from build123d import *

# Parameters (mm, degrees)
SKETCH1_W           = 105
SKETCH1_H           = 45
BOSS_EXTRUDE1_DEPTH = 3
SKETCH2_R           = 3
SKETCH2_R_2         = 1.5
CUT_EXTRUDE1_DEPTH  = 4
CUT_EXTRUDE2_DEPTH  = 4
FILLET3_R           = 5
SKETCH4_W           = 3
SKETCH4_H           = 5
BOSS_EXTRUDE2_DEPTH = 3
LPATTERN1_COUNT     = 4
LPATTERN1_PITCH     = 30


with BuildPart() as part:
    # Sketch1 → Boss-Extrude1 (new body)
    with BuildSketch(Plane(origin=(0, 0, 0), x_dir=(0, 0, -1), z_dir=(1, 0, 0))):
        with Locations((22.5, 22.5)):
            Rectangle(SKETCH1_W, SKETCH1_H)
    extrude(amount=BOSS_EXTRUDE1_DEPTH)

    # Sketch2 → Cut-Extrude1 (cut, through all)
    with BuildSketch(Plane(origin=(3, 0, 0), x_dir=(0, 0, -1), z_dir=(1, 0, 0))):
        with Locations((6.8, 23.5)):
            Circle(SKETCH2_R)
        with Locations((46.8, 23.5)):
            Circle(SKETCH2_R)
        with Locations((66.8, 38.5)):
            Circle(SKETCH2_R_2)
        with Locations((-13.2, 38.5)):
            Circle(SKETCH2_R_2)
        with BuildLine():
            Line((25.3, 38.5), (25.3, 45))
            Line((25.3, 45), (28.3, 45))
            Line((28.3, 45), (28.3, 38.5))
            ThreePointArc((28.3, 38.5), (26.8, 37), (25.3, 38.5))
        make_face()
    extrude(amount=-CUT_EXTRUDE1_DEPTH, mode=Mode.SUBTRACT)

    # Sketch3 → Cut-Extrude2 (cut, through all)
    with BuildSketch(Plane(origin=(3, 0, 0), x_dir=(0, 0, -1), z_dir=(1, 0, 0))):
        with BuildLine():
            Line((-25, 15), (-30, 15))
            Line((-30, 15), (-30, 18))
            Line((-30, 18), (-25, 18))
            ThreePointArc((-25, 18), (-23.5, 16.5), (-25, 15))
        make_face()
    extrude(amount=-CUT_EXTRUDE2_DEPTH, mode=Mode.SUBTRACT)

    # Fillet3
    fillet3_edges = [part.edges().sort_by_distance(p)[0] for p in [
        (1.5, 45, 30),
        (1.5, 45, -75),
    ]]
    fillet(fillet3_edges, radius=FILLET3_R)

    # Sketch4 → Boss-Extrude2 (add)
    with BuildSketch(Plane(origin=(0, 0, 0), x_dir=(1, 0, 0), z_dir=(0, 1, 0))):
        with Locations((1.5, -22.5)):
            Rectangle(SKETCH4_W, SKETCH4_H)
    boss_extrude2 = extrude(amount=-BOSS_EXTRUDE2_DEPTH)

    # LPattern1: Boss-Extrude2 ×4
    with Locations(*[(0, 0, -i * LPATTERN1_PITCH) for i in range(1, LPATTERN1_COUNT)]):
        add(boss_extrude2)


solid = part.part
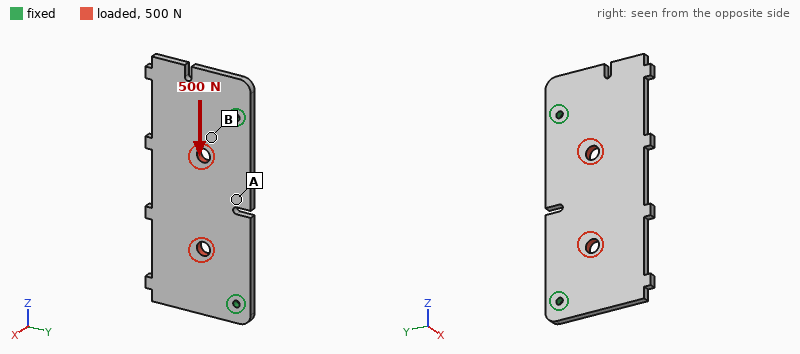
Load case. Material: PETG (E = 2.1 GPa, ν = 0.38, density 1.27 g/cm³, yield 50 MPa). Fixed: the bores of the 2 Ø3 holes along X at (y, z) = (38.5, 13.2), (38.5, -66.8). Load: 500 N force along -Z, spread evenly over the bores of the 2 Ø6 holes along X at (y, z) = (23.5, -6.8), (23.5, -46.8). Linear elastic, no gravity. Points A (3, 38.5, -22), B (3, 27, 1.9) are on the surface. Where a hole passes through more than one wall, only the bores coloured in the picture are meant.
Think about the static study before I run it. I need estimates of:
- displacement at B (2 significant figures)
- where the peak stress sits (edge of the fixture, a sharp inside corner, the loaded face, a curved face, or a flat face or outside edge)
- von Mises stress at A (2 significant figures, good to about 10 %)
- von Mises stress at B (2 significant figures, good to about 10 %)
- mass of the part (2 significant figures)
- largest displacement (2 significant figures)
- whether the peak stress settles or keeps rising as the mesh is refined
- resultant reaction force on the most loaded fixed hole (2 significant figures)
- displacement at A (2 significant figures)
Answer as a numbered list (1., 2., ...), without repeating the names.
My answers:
1. 0.060 mm
2. edge of the fixture
3. 2.0 MPa
4. 4.2 MPa
5. 18 g
6. 0.10 mm
7. keeps rising
8. 270 N
9. 0.055 mm
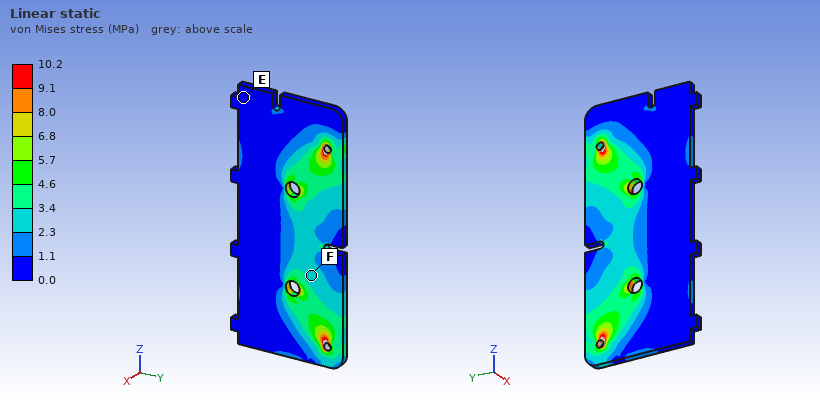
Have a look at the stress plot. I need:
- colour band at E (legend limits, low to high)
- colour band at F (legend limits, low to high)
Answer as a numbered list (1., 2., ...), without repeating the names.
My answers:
1. 0.0 to 1.1 MPa
2. 2.3 to 3.4 MPa
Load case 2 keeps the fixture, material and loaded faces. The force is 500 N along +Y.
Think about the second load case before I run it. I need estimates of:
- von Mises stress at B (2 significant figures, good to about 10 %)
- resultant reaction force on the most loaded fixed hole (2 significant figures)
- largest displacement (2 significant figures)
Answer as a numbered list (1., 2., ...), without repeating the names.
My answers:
1. 5.0 MPa
2. 290 N
3. 0.15 mm
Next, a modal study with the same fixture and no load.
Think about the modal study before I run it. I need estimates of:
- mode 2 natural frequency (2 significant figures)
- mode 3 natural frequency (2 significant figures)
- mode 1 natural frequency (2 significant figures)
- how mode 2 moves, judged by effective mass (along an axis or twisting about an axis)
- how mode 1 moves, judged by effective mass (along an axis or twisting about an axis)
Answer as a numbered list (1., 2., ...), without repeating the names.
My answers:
1. 470 Hz
2. 580 Hz
3. 260 Hz
4. twisting about Y
5. along X
